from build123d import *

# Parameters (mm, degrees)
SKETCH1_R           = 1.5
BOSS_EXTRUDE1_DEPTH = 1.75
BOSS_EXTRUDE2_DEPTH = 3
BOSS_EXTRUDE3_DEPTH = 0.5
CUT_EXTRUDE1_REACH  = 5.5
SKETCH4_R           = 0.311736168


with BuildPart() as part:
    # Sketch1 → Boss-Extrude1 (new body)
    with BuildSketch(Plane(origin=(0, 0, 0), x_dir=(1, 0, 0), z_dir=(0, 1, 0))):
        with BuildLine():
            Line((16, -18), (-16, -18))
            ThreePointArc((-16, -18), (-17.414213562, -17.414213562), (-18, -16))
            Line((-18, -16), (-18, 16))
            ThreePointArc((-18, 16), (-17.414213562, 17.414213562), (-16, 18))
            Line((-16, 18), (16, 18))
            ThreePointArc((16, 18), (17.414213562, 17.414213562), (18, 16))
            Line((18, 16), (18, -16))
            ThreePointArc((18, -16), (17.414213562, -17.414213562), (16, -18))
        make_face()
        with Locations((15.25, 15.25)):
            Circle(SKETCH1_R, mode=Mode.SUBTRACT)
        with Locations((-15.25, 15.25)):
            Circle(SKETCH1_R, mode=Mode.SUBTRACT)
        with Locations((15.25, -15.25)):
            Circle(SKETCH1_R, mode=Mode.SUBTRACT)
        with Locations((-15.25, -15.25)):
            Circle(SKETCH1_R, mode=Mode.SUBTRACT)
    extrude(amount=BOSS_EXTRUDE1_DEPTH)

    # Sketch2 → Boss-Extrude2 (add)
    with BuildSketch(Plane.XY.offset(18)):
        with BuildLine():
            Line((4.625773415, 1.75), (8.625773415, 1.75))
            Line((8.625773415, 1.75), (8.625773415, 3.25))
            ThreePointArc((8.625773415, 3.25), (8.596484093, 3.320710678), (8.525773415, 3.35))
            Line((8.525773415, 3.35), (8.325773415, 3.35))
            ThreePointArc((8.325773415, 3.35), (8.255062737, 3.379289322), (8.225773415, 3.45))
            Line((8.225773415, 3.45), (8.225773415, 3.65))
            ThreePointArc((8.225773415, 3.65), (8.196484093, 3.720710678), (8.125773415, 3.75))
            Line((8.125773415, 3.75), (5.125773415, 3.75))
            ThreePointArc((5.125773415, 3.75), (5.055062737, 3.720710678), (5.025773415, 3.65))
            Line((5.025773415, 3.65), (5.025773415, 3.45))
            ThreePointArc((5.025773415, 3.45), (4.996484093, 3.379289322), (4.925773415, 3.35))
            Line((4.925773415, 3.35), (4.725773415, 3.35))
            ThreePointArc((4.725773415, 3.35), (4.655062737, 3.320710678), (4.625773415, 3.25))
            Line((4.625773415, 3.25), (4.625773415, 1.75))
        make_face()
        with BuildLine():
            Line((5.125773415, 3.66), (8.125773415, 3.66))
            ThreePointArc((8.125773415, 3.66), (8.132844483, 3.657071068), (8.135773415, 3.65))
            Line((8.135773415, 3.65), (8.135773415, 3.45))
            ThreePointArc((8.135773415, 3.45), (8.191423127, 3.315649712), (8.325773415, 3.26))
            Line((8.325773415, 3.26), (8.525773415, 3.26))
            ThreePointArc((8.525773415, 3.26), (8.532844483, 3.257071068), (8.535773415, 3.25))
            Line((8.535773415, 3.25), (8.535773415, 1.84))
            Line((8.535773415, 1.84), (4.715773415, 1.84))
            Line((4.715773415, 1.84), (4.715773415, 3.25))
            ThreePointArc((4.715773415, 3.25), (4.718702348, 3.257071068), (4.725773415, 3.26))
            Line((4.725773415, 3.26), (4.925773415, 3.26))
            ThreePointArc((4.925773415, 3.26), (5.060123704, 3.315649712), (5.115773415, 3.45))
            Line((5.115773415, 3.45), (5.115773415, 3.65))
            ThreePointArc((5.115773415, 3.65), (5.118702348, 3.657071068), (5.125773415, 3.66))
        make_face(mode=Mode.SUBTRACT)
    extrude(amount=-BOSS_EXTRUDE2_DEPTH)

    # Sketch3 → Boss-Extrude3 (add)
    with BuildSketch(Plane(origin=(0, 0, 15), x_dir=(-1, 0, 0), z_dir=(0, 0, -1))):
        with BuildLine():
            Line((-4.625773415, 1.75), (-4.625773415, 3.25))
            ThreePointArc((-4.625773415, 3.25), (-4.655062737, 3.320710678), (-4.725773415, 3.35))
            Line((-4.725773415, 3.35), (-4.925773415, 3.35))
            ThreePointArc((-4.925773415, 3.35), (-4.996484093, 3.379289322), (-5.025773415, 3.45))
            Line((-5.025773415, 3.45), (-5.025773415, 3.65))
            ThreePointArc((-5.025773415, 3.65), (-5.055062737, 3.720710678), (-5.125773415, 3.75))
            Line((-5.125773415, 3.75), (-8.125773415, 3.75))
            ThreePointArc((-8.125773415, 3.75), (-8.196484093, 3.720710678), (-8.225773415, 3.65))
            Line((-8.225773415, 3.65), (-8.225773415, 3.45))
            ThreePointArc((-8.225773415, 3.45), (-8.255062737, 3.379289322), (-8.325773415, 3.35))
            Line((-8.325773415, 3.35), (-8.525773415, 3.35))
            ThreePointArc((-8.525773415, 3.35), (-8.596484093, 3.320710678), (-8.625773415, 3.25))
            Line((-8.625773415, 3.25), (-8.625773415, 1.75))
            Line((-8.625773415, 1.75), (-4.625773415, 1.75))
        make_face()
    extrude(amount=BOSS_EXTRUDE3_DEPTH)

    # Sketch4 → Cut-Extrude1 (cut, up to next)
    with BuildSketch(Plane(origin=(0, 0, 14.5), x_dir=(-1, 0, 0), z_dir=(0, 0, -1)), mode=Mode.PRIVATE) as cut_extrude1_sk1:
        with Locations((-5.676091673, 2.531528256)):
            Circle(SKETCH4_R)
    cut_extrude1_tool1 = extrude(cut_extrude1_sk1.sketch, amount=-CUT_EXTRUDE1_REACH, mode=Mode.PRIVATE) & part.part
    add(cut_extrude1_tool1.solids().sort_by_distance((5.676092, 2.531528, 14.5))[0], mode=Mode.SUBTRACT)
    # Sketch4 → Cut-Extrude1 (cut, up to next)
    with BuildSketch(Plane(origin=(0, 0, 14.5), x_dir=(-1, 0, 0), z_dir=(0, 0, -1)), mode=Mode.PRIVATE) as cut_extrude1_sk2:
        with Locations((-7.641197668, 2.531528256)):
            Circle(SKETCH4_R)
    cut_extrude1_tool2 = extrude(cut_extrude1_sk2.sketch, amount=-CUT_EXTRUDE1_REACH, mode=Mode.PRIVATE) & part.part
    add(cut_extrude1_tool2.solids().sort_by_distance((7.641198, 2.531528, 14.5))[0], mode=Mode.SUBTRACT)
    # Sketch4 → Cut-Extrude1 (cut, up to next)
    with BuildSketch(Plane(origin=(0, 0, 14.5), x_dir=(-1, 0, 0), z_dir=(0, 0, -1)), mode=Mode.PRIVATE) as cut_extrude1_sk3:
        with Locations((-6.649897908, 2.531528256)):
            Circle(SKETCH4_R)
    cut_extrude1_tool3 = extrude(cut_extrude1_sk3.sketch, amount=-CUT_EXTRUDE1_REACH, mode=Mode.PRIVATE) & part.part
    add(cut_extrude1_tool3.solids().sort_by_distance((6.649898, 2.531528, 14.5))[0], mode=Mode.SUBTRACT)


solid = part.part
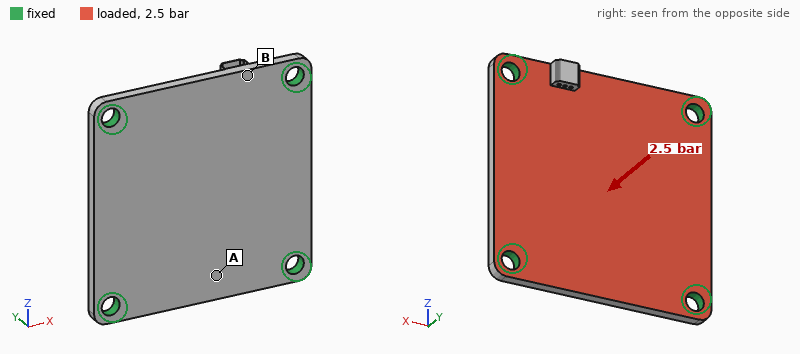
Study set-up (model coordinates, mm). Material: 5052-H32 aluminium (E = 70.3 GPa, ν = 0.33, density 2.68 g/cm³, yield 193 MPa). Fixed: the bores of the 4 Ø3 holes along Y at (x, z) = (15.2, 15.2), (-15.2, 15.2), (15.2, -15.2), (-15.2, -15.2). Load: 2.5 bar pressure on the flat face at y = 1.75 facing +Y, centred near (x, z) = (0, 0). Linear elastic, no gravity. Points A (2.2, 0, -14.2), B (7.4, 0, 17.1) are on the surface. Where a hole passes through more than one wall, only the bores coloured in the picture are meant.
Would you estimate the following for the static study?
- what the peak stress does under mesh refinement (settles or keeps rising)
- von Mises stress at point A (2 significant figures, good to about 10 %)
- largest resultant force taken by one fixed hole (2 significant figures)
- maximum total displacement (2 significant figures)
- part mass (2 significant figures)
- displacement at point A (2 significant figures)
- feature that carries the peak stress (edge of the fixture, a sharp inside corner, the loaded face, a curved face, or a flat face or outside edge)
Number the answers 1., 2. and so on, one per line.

1. keeps rising
2. 21 MPa
3. 79 N
4. 40 µm
5. 5.9 g
6. 22 µm
7. edge of the fixture
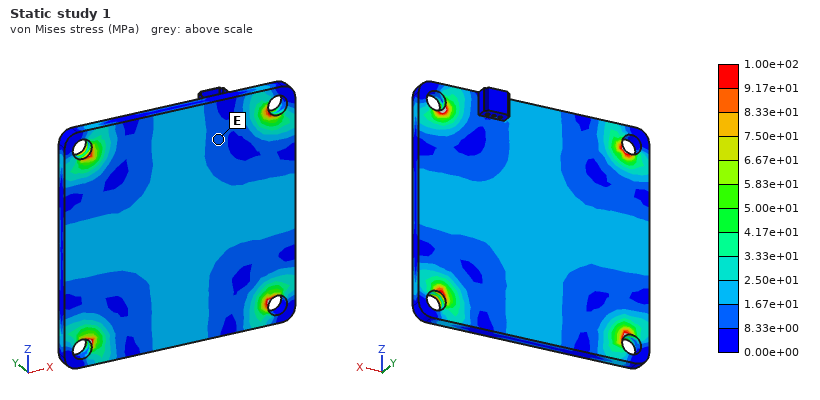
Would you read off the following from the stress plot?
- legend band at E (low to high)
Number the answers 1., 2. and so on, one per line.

1. 8.33e+00 to 1.67e+01 MPa
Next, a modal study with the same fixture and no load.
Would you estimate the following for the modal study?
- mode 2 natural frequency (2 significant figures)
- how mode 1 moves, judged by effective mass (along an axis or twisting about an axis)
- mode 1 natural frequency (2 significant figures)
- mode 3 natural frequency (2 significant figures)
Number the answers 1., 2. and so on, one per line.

1. 12 kHz
2. along Y
3. 7100 Hz
4. 12 kHz
